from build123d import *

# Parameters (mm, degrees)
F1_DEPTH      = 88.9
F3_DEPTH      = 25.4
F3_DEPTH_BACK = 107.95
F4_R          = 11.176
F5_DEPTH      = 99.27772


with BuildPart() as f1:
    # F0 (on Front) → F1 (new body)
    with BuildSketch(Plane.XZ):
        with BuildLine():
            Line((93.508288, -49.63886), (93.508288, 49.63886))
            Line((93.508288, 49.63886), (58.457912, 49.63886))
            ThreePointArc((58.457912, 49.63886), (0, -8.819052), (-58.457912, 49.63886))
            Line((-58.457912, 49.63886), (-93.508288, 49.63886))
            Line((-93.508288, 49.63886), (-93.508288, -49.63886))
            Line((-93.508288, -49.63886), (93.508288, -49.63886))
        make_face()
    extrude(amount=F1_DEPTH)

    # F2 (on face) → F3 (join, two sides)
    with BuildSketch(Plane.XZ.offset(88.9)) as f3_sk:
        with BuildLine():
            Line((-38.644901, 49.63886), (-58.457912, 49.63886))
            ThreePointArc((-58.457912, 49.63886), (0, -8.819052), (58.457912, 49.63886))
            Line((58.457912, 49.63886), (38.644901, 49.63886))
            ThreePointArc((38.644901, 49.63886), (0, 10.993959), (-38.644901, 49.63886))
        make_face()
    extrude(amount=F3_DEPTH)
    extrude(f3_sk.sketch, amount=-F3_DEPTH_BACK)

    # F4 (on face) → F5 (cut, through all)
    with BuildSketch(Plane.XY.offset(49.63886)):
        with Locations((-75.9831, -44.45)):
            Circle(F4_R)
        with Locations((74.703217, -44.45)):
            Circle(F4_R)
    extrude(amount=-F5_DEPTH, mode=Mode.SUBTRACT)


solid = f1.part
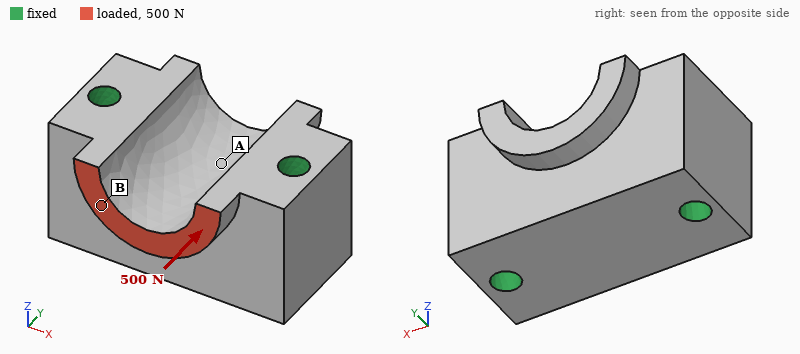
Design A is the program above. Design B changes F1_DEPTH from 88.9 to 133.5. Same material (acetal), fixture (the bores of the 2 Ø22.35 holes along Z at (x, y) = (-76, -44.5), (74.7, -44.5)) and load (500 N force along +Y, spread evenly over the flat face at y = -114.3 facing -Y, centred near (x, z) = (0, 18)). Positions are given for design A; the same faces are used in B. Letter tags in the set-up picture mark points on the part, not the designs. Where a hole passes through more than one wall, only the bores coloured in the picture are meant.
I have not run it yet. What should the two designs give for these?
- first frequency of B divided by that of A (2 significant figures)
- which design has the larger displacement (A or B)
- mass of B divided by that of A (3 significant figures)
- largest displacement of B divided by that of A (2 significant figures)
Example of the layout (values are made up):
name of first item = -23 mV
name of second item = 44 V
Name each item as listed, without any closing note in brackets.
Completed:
first frequency of B divided by that of A = 0.74
which design has the larger displacement = A
mass of B divided by that of A = 1.39
largest displacement of B divided by that of A = 0.71
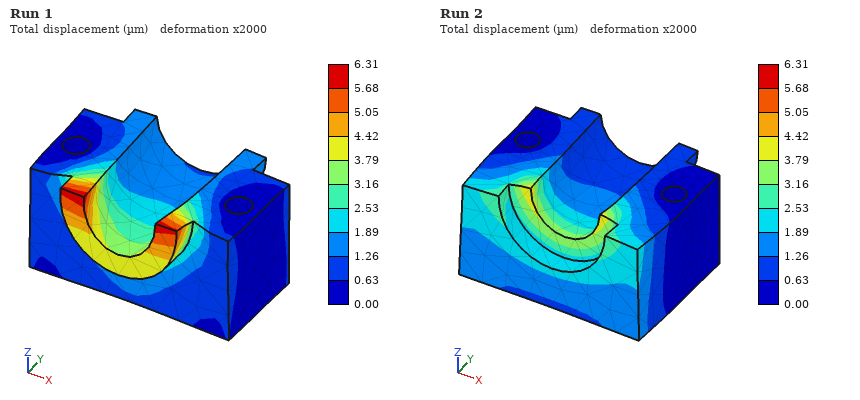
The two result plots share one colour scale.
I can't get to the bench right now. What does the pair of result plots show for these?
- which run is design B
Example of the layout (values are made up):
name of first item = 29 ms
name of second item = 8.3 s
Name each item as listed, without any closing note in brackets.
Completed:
which run is design B = Run 2
